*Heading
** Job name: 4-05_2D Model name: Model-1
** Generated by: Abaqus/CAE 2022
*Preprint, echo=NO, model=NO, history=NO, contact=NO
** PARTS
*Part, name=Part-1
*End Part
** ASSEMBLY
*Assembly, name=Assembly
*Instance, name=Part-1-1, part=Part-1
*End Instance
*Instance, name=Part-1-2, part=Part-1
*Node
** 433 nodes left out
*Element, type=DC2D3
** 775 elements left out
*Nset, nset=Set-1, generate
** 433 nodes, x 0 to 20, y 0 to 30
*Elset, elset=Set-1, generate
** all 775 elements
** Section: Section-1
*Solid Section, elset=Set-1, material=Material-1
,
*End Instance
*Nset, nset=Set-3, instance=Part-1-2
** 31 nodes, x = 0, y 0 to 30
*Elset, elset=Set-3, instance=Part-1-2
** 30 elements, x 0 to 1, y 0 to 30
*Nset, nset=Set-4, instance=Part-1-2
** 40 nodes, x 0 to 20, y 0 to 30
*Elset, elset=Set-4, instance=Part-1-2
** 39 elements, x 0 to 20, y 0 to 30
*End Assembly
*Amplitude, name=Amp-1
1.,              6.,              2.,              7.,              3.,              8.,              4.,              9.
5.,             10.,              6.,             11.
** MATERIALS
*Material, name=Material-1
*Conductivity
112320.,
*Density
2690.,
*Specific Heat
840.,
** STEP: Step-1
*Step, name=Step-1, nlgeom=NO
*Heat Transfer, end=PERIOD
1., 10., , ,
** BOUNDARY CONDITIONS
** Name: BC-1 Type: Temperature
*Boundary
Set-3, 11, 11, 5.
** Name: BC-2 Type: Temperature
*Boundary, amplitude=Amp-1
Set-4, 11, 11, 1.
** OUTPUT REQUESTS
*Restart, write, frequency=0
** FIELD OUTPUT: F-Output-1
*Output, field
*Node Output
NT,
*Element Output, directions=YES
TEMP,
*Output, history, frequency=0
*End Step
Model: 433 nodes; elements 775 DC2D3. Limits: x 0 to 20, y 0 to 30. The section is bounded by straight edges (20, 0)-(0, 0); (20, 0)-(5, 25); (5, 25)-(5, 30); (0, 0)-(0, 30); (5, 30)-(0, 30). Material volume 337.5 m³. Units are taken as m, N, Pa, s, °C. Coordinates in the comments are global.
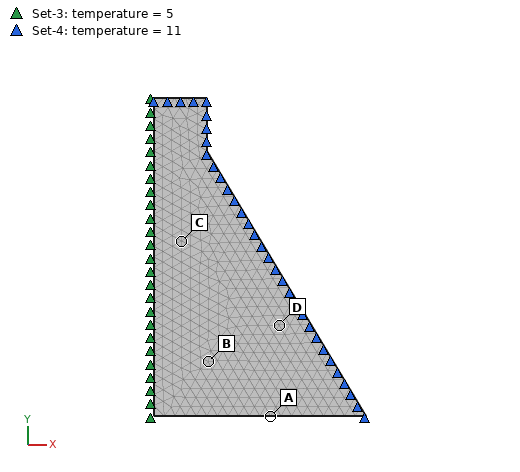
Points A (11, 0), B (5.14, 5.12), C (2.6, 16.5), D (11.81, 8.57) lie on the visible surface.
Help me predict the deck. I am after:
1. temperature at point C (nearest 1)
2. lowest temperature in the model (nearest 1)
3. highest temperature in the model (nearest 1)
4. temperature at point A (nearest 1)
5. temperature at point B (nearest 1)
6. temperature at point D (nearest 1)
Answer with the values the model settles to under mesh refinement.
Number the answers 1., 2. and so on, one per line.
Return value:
1. 0 °C
2. 0 °C
3. 11 °C
4. 0 °C
5. 0 °C
6. 0 °C
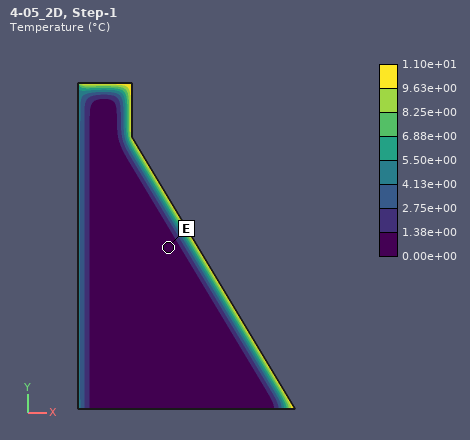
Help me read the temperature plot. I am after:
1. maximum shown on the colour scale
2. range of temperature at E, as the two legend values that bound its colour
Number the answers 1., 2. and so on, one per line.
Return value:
1. 1.10e+01 °C
2. 0.00e+00 to 1.38e+00 °C
